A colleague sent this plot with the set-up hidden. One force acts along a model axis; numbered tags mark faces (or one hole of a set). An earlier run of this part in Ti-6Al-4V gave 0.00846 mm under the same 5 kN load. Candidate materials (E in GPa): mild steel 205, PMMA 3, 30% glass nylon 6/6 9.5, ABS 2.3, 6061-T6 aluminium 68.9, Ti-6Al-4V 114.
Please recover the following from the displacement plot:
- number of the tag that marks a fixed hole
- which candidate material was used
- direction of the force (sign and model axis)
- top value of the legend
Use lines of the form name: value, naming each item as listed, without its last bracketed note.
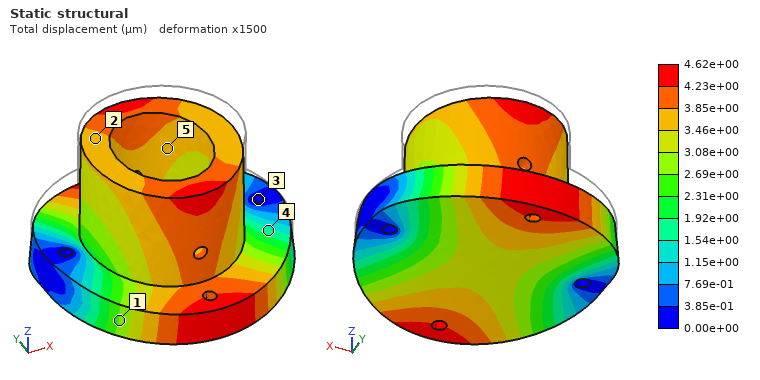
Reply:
number of the tag that marks a fixed hole: 3
which candidate material was used: mild steel
direction of the force: -Z
top value of the legend: 4.62e+00 µm
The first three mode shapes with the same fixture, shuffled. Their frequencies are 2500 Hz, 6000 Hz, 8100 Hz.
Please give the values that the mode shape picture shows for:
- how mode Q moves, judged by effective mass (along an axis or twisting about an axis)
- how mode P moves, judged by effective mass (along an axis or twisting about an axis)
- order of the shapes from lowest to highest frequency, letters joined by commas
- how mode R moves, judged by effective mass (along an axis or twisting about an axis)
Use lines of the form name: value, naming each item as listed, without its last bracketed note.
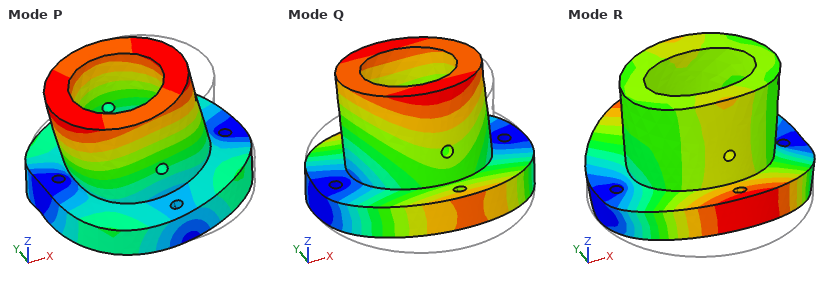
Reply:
how mode Q moves, judged by effective mass: along Y
how mode P moves, judged by effective mass: along X
order of the shapes from lowest to highest frequency, letters joined by commas: Q, R, P
how mode R moves, judged by effective mass: along Z
